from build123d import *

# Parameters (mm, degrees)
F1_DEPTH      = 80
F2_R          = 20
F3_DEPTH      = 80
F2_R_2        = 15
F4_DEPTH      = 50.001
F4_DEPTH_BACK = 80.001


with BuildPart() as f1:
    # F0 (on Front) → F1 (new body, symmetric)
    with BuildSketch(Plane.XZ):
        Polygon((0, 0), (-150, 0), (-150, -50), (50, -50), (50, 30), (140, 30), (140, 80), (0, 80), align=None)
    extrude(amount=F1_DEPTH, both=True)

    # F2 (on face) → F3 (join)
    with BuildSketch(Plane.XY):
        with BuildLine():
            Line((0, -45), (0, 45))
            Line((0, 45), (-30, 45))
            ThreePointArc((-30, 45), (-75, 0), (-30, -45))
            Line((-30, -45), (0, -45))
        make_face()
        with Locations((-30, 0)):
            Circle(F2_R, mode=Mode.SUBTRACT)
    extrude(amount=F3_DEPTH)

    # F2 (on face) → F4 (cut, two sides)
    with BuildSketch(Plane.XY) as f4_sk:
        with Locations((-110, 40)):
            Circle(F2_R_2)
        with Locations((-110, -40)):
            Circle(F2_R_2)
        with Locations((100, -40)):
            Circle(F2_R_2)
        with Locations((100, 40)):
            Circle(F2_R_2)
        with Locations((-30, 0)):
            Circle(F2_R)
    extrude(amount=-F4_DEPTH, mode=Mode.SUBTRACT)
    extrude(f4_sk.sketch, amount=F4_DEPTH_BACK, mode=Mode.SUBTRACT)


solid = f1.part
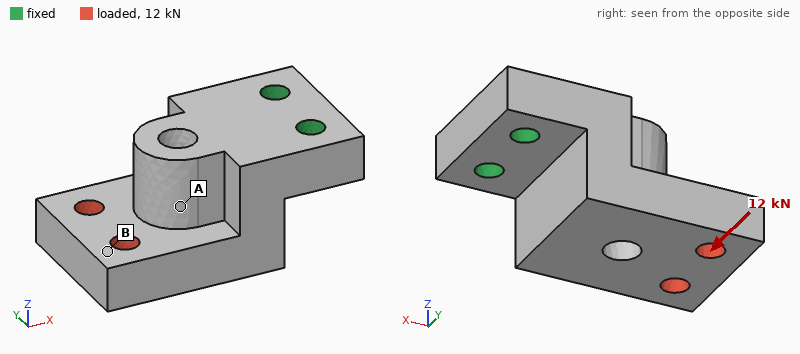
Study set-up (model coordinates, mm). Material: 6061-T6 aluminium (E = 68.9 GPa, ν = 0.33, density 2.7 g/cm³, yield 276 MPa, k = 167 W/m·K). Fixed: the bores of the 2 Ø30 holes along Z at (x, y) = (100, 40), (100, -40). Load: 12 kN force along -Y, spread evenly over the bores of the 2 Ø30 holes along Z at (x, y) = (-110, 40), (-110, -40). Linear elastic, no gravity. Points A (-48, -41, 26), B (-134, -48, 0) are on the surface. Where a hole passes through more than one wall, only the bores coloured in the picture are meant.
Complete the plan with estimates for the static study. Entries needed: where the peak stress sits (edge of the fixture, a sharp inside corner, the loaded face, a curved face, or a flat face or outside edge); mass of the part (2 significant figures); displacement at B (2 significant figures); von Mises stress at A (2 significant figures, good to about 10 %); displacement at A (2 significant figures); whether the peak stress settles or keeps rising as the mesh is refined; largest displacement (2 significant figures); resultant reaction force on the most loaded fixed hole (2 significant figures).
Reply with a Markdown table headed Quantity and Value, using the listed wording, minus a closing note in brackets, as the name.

| Quantity | Value |
|---|---|
| where the peak stress sits | edge of the fixture |
| mass of the part | 8.4 kg |
| displacement at B | 79 µm |
| von Mises stress at A | 3.8 MPa |
| displacement at A | 38 µm |
| whether the peak stress settles or keeps rising as the mesh is refined | keeps rising |
| largest displacement | 94 µm |
| resultant reaction force on the most loaded fixed hole | 27 kN |
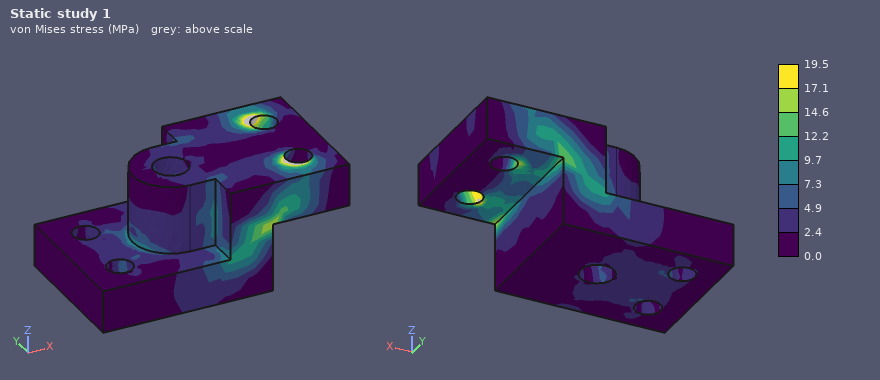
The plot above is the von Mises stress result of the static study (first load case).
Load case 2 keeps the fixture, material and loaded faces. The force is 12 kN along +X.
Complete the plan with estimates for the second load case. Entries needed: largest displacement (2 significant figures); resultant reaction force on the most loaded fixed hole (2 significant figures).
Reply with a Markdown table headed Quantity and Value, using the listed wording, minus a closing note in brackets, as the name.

| Quantity | Value |
|---|---|
| largest displacement | 0.14 mm |
| resultant reaction force on the most loaded fixed hole | 6.1 kN |
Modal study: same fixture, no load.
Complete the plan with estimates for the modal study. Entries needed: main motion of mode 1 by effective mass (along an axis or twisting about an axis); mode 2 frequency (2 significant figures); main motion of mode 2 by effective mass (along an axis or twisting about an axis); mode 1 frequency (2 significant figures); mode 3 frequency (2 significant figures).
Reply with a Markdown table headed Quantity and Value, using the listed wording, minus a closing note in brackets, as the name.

| Quantity | Value |
|---|---|
| main motion of mode 1 by effective mass | along Z |
| mode 2 frequency | 1200 Hz |
| main motion of mode 2 by effective mass | along Y |
| mode 1 frequency | 610 Hz |
| mode 3 frequency | 2000 Hz |
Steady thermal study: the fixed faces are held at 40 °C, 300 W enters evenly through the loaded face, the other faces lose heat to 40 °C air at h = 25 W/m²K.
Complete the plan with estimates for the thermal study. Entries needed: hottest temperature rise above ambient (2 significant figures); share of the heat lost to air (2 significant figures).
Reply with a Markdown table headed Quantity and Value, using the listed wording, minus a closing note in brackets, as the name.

| Quantity | Value |
|---|---|
| hottest temperature rise above ambient | 41 K |
| share of the heat lost to air | 27 % |
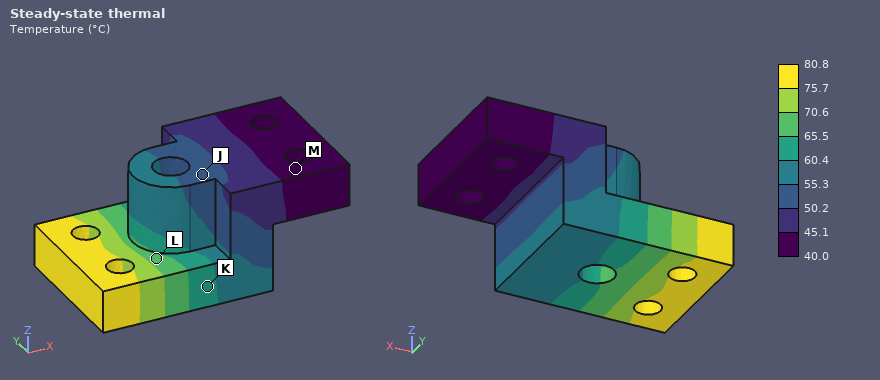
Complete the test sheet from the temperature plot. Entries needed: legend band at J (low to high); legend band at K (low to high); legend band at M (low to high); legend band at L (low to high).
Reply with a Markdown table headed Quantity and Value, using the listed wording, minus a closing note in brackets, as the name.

| Quantity | Value |
|---|---|
| legend band at J | 50.2 to 55.3 °C |
| legend band at K | 60.4 to 65.5 °C |
| legend band at M | 40.0 to 45.1 °C |
| legend band at L | 65.5 to 70.6 °C |
